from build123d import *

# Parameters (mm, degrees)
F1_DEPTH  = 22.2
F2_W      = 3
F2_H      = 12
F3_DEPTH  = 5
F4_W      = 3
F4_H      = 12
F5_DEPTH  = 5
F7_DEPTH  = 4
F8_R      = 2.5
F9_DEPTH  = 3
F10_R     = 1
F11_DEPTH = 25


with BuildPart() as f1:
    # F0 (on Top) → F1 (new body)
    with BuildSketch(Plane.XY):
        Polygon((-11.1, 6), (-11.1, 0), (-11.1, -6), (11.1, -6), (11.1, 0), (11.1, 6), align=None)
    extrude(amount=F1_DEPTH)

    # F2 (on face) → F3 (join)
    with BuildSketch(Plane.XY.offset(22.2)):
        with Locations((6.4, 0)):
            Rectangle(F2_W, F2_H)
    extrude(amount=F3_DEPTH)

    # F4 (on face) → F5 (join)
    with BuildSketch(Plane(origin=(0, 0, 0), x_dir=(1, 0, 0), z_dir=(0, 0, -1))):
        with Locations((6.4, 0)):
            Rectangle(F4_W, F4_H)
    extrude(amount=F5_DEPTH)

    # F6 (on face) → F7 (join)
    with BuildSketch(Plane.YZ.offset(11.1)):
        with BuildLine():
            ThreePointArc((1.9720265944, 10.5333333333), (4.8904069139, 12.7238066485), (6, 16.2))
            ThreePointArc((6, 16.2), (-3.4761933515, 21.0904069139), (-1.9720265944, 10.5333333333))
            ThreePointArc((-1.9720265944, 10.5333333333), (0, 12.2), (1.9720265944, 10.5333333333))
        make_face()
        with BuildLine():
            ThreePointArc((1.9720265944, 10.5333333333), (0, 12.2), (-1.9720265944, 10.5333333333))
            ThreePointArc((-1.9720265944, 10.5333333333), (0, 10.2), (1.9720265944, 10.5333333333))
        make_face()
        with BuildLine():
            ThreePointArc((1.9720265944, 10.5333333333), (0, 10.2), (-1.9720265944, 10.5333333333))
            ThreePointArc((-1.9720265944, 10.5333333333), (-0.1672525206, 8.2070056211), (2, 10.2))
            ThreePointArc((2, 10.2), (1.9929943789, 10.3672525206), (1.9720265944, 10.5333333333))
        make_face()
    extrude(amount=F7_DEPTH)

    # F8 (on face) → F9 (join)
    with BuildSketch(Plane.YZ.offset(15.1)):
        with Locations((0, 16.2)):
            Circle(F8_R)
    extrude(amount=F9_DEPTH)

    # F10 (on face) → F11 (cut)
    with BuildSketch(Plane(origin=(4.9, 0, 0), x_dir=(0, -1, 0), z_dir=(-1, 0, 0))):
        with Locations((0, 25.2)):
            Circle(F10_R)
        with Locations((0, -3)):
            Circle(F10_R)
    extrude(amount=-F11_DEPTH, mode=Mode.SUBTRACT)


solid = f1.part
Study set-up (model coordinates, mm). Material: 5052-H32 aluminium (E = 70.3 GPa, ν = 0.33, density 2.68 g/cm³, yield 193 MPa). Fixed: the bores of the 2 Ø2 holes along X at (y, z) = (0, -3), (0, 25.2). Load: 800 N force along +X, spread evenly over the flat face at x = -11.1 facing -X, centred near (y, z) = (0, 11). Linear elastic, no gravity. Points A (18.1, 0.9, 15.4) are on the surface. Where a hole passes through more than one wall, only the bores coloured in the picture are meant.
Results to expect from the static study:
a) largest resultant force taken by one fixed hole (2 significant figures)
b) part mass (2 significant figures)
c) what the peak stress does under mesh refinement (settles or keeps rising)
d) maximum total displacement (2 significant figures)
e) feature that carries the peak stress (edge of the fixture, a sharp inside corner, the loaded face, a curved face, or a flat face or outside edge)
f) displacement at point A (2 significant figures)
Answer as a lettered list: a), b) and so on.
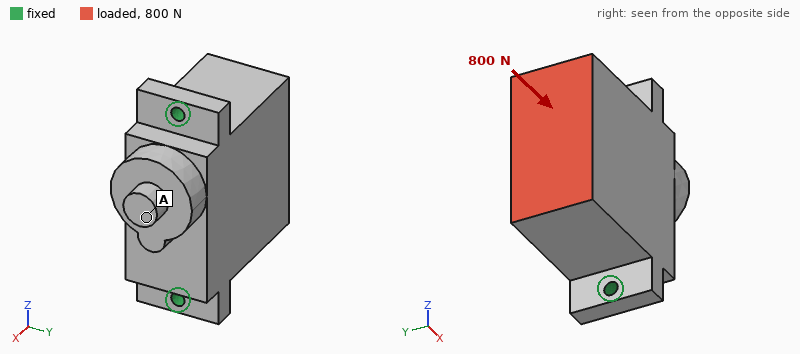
a) 400 N
b) 18 g
c) keeps rising
d) 5.3 µm
e) edge of the fixture
f) 4.7 µm
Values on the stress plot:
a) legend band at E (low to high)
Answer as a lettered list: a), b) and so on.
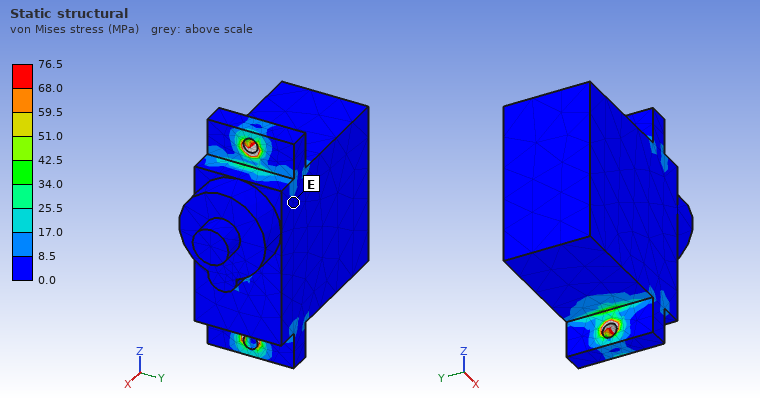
a) 0.0 to 8.5 MPa
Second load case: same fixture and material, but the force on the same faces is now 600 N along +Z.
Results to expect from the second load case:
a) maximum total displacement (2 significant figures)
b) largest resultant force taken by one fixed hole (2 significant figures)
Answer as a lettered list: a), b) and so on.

a) 11 µm
b) 510 N
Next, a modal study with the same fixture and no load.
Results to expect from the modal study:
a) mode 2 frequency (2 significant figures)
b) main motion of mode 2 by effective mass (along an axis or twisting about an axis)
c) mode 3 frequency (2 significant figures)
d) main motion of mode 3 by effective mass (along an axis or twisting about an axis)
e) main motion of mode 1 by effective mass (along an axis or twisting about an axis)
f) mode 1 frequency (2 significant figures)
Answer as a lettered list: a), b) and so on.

a) 16 kHz
b) along X
c) 17 kHz
d) along Z
e) along Y
f) 4400 Hz
